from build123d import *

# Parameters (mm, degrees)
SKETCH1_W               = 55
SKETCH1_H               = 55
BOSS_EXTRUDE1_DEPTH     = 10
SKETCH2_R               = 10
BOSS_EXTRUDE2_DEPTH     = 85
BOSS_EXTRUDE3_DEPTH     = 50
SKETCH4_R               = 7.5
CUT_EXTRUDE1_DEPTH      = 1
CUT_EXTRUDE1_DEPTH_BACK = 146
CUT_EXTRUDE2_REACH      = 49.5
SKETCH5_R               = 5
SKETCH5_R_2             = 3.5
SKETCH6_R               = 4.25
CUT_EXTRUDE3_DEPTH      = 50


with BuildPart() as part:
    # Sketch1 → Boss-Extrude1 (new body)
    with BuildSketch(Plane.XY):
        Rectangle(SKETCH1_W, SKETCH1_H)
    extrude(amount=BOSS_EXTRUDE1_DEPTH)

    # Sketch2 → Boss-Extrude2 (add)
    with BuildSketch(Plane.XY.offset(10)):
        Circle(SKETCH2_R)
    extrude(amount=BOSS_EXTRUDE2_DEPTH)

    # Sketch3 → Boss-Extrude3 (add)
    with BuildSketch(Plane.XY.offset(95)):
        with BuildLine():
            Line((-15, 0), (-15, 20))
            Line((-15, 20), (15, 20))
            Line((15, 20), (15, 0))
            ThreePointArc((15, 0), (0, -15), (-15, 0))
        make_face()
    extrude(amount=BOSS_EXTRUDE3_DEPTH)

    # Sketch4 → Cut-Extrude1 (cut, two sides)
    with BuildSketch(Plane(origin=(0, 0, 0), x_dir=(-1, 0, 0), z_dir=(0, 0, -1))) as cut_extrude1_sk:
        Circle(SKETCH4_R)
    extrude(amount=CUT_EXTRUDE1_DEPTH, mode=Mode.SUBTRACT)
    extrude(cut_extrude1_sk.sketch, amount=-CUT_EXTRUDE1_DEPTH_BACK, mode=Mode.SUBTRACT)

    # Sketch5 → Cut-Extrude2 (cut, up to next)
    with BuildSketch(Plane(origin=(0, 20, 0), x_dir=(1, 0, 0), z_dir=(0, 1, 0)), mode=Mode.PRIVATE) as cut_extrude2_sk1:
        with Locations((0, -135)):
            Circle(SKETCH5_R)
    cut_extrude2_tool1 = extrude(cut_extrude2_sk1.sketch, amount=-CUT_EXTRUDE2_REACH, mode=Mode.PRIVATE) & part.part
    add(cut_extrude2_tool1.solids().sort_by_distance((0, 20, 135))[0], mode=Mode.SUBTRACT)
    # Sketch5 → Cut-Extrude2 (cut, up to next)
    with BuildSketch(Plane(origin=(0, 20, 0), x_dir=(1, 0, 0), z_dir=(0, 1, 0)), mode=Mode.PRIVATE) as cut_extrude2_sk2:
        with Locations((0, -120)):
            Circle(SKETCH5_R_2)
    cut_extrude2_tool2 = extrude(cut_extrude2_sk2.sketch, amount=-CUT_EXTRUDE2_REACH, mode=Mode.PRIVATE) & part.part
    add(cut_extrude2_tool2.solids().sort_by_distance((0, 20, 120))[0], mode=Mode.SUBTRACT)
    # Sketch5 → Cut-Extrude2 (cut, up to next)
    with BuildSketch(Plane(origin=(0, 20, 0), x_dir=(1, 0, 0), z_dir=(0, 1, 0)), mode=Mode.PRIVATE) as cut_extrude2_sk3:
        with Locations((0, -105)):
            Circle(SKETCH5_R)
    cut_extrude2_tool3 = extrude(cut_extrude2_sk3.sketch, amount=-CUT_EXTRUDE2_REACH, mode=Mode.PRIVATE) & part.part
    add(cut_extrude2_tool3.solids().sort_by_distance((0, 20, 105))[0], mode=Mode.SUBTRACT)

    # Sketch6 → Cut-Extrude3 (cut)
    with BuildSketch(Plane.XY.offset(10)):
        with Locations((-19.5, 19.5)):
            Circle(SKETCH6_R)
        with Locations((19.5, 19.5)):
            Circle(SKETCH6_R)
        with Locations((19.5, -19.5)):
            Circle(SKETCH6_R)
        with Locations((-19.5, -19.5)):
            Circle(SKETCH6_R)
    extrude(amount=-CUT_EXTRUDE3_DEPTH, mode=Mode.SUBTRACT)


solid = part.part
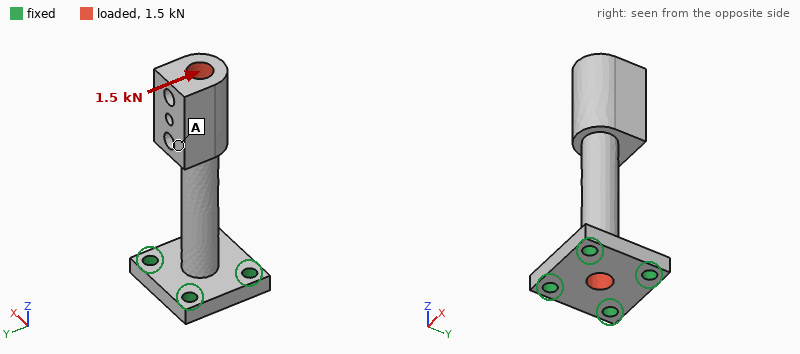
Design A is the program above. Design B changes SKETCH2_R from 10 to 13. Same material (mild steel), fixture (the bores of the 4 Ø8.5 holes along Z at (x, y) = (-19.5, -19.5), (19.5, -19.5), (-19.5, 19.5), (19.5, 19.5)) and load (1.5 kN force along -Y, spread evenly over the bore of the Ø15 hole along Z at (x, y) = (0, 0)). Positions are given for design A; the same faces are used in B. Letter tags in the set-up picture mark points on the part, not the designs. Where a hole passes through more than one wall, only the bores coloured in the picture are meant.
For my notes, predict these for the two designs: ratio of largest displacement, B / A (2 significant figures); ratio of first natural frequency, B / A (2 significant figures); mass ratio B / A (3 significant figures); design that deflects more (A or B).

0.31
1.8
1.25
A
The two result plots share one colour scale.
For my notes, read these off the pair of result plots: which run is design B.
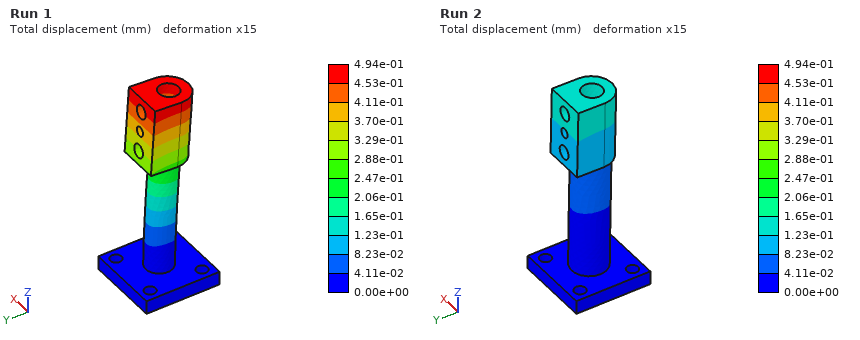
Run 2
